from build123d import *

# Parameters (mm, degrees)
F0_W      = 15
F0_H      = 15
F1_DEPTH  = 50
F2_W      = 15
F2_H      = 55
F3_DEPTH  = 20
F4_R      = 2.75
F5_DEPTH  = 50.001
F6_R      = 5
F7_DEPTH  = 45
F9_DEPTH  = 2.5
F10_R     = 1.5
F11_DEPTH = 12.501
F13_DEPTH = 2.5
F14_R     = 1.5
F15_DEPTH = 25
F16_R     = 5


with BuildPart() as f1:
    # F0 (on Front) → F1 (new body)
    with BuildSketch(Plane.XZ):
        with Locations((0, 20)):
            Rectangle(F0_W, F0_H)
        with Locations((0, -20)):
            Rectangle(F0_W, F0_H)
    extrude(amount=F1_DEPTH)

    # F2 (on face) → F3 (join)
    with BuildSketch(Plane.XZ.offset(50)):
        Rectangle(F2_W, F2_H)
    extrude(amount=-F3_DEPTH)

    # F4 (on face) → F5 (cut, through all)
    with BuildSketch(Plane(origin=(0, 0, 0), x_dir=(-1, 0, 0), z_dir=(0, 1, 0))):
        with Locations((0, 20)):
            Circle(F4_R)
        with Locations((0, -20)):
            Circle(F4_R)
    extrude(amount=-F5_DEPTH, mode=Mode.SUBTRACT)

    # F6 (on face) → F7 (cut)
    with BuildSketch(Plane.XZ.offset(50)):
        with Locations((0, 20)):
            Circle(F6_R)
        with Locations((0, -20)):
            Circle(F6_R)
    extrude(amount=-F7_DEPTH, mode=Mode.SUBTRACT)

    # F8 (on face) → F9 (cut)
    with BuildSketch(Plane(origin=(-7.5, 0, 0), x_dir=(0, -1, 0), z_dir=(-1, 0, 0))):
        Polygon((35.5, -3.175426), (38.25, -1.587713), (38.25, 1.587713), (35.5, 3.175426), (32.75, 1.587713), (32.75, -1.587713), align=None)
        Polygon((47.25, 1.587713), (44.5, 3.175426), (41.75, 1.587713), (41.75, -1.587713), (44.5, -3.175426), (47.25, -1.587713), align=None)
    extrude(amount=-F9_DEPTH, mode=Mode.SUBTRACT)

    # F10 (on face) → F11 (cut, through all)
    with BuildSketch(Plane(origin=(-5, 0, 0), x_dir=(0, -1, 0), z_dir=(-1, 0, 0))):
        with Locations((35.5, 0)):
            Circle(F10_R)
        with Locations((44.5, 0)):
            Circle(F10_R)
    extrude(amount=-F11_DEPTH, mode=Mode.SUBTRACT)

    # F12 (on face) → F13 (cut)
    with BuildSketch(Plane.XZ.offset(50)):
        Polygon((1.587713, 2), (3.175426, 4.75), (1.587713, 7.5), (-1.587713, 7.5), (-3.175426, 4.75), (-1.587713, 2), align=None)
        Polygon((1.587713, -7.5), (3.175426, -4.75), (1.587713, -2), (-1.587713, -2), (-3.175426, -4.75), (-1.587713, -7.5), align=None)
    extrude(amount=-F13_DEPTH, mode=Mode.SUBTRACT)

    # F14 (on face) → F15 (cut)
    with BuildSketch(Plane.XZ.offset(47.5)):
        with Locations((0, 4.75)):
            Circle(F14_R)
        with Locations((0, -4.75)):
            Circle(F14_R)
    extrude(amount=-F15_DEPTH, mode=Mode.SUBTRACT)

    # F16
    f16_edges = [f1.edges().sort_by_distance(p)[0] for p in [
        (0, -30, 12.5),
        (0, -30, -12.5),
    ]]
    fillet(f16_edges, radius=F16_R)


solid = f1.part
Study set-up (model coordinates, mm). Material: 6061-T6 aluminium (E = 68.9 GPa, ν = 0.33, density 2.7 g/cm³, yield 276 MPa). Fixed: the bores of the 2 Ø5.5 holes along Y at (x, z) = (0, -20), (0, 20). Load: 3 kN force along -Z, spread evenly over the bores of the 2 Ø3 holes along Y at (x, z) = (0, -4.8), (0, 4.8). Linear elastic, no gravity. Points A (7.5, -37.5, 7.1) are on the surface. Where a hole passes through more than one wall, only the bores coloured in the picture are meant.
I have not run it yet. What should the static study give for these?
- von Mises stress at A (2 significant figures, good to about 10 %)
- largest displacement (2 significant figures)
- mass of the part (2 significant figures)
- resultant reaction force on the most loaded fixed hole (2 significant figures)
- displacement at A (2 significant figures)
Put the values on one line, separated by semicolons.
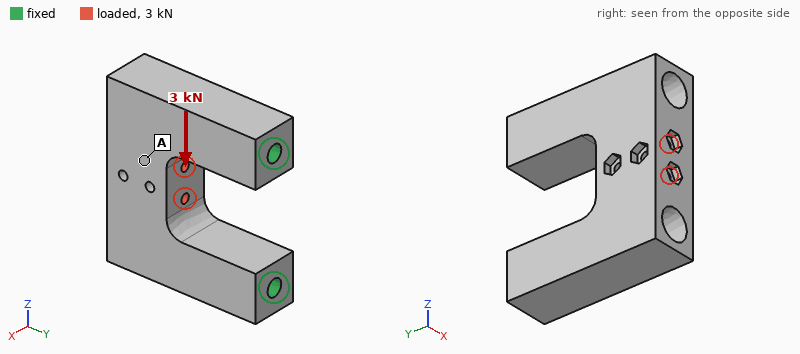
19 MPa; 81 µm; 60 g; 2.4 kN; 70 µm
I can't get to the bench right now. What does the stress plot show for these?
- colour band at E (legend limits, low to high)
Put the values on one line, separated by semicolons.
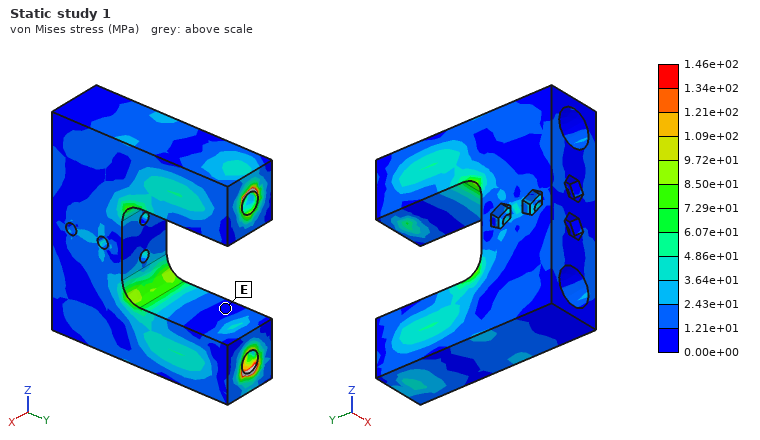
0.00e+00 to 1.21e+01 MPa
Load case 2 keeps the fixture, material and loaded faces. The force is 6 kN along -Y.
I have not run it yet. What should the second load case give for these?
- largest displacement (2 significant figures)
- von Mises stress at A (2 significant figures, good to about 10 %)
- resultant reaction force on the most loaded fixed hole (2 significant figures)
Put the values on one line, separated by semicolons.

27 µm; 22 MPa; 3.1 kN
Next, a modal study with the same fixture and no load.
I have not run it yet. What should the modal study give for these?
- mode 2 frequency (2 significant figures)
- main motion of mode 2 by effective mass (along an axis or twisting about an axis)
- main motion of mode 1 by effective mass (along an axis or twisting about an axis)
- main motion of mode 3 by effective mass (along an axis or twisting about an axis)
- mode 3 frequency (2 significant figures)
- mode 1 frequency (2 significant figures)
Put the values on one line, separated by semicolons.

5000 Hz; along Z; along X; twisting about Y; 6200 Hz; 2500 Hz
